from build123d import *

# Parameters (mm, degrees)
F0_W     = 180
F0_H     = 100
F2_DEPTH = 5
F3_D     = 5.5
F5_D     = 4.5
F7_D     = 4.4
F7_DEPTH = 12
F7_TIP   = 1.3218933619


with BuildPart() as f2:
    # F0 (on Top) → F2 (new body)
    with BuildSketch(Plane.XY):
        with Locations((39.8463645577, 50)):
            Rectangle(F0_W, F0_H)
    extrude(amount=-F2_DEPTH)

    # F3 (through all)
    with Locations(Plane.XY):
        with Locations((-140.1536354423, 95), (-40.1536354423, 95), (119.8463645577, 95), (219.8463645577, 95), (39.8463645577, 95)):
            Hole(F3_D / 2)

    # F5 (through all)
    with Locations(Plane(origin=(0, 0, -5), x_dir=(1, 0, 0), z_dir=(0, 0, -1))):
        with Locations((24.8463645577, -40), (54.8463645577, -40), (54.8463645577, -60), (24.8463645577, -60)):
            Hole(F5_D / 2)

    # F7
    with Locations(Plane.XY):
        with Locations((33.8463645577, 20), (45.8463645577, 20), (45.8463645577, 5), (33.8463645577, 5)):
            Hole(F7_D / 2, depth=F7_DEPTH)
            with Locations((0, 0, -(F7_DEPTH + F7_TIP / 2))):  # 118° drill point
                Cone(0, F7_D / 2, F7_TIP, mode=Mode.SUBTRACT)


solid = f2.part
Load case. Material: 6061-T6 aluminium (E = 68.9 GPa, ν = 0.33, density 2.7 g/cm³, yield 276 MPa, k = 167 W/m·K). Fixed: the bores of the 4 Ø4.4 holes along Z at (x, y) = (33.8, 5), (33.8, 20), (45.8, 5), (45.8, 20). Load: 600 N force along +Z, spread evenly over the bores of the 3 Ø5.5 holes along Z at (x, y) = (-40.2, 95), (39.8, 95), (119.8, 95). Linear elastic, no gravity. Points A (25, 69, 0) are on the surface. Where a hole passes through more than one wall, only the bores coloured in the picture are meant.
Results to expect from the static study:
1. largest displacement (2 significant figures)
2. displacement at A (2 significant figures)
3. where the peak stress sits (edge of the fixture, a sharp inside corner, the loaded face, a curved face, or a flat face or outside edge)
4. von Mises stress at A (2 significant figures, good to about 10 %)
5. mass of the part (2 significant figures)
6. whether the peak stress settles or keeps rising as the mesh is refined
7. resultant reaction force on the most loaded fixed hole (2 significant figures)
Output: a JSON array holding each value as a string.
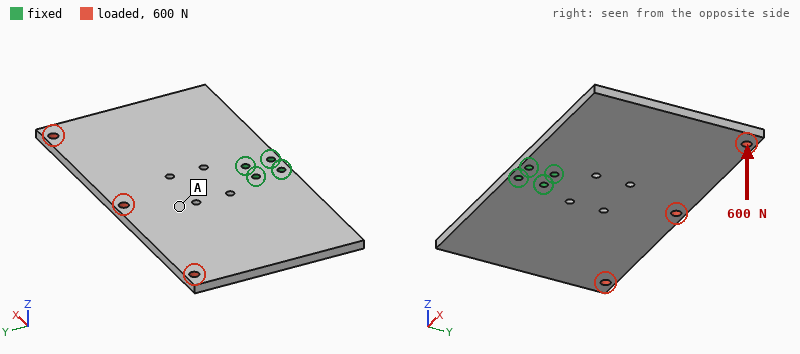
["1.7 mm", "0.63 mm", "edge of the fixture", "32 MPa", "240 g", "keeps rising", "1.0 kN"]
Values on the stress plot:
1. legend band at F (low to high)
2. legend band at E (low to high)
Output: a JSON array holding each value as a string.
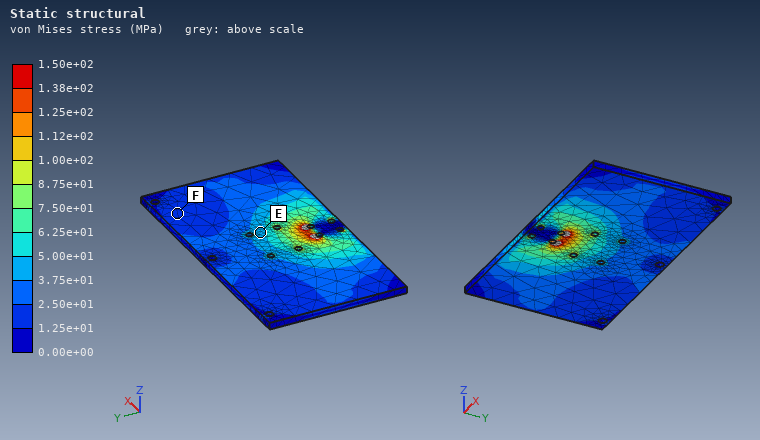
["1.25e+01 to 2.50e+01 MPa", "3.75e+01 to 5.00e+01 MPa"]
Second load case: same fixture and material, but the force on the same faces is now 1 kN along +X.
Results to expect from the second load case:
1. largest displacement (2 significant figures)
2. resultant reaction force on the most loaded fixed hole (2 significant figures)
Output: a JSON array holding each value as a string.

["87 µm", "2.4 kN"]
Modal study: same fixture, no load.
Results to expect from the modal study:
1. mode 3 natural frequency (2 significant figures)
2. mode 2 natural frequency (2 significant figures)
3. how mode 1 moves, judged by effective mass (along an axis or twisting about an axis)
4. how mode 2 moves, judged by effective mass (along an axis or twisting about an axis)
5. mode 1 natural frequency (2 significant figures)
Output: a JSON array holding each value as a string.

["680 Hz", "420 Hz", "twisting about Y", "along Z", "360 Hz"]
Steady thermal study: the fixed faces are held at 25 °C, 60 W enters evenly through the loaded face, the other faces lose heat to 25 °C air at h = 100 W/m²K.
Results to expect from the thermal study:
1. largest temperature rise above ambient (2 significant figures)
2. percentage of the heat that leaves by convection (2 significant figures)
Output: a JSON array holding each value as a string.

["37 K", "73 %"]
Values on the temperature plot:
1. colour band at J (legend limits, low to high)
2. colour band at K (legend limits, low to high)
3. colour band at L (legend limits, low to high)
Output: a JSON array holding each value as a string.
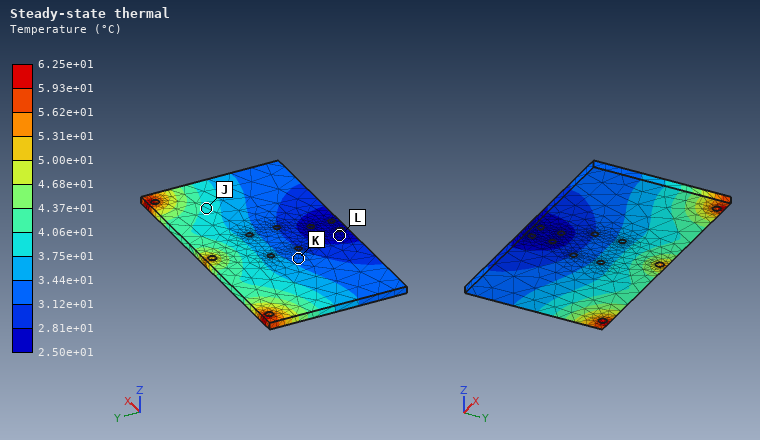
["3.75e+01 to 4.06e+01 °C", "3.12e+01 to 3.44e+01 °C", "2.50e+01 to 2.81e+01 °C"]
